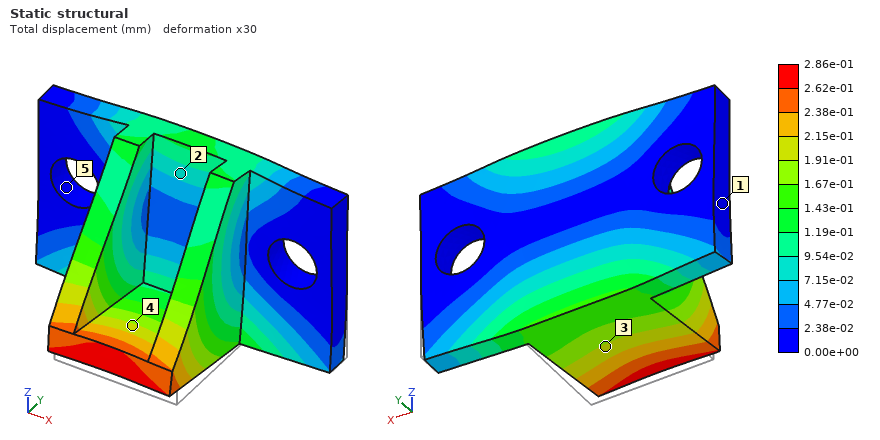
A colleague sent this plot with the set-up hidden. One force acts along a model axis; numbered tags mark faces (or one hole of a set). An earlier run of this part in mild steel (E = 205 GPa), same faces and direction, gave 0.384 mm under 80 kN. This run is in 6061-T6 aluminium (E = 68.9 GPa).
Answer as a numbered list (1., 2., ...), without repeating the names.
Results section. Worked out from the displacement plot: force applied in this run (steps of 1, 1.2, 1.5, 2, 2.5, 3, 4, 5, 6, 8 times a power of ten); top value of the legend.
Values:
1. 20 kN
2. 2.86e-01 mm
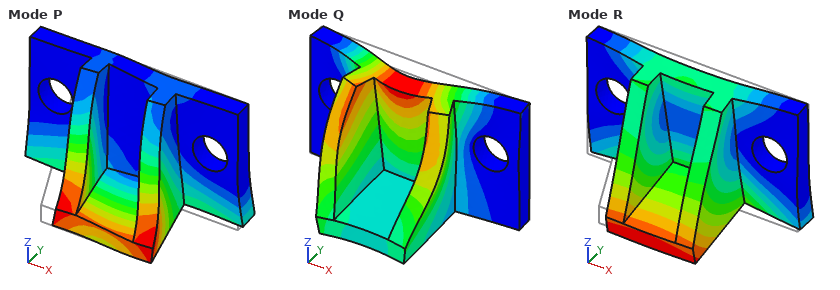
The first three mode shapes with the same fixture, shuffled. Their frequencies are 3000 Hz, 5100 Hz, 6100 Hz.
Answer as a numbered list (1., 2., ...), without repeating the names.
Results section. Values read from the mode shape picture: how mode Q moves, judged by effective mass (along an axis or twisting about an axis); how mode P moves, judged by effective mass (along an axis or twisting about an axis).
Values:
1. along Y
2. along X
